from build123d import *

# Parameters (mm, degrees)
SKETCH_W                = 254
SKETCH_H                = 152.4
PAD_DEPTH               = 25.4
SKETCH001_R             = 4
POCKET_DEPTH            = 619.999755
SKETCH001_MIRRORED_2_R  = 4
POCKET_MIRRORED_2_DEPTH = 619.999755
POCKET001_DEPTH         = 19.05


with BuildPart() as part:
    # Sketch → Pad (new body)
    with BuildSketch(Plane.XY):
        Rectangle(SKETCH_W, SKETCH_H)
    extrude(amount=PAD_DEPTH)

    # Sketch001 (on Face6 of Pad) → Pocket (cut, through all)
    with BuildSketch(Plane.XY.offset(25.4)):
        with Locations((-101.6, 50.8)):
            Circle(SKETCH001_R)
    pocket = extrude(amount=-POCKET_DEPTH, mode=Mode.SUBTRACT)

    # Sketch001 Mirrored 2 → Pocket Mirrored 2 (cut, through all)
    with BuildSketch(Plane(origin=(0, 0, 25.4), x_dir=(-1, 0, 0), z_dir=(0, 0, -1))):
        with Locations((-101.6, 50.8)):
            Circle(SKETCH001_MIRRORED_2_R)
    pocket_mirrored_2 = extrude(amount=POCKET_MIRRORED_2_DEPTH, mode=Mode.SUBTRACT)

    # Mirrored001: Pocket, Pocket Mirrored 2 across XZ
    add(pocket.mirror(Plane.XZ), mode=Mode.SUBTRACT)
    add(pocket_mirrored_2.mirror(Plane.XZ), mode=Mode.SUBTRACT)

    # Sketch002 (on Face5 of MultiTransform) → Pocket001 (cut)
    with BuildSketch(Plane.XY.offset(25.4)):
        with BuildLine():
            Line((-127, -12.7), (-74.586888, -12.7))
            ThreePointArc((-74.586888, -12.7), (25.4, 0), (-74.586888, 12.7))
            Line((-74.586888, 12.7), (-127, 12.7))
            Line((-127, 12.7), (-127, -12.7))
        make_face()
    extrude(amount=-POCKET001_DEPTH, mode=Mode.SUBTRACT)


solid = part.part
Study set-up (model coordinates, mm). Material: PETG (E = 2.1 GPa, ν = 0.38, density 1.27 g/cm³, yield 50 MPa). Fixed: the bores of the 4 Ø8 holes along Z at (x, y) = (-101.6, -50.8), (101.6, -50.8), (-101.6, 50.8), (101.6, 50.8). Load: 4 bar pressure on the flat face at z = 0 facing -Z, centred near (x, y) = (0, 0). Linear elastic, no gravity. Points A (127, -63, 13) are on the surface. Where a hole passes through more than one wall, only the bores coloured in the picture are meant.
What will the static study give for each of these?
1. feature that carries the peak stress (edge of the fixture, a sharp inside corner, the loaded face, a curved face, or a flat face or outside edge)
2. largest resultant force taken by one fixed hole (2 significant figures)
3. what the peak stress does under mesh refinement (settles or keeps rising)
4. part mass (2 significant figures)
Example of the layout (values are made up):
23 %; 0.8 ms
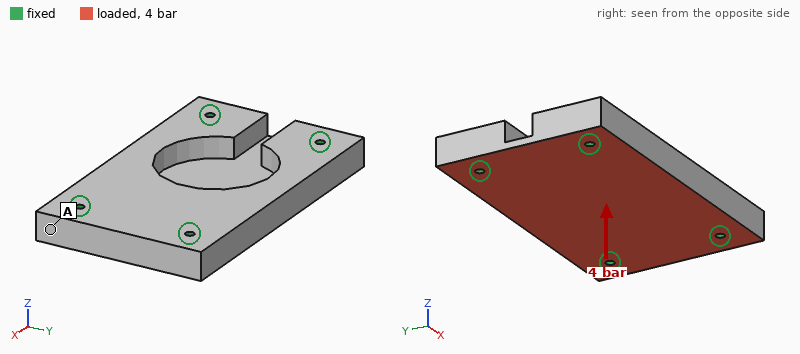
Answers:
edge of the fixture; 4.1 kN; keeps rising; 1.0 kg
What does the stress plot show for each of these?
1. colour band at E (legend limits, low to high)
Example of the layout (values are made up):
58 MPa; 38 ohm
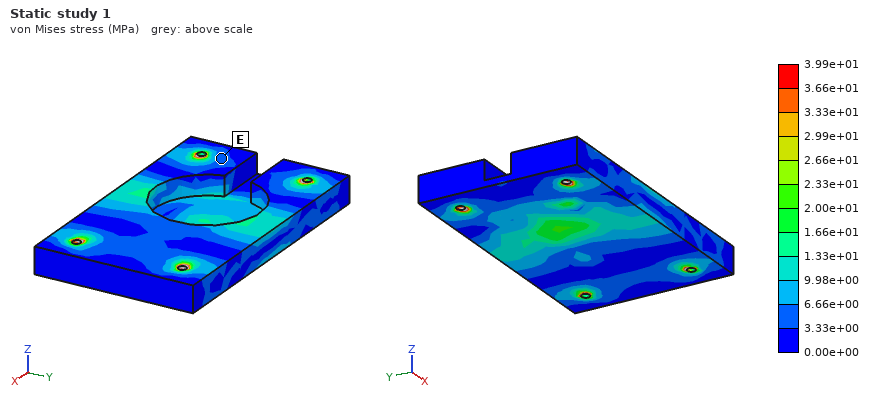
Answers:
3.33e+00 to 6.66e+00 MPa
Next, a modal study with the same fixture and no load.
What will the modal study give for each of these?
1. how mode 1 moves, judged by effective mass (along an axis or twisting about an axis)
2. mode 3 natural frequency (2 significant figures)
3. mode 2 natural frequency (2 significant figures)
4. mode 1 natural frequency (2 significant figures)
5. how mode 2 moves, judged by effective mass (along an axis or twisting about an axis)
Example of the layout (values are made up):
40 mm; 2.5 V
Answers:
along Z; 1300 Hz; 830 Hz; 640 Hz; twisting about X
